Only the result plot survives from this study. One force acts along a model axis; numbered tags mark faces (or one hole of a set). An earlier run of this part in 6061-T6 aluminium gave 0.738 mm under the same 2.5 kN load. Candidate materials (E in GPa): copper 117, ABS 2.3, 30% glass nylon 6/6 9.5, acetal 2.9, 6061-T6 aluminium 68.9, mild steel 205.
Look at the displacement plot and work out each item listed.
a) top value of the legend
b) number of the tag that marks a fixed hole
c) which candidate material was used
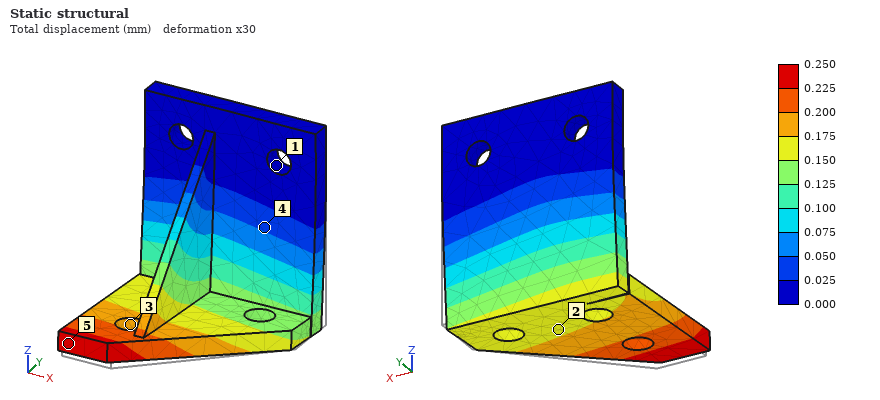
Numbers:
0.250 mm
1
mild steel
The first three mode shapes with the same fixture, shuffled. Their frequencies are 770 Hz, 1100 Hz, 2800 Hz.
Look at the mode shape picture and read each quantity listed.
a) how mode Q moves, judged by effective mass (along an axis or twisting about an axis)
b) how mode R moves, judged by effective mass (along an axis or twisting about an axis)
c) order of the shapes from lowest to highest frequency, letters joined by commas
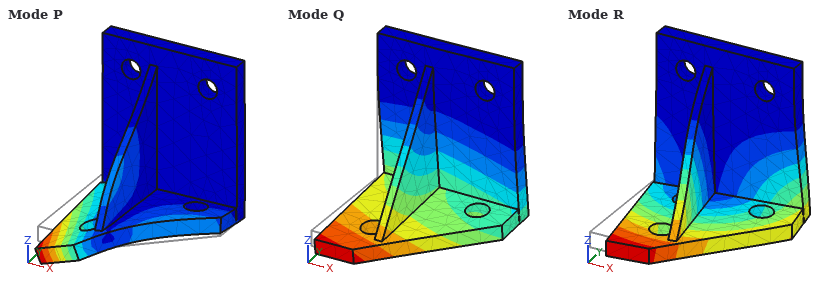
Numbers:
along Y
along X
Q, R, P
